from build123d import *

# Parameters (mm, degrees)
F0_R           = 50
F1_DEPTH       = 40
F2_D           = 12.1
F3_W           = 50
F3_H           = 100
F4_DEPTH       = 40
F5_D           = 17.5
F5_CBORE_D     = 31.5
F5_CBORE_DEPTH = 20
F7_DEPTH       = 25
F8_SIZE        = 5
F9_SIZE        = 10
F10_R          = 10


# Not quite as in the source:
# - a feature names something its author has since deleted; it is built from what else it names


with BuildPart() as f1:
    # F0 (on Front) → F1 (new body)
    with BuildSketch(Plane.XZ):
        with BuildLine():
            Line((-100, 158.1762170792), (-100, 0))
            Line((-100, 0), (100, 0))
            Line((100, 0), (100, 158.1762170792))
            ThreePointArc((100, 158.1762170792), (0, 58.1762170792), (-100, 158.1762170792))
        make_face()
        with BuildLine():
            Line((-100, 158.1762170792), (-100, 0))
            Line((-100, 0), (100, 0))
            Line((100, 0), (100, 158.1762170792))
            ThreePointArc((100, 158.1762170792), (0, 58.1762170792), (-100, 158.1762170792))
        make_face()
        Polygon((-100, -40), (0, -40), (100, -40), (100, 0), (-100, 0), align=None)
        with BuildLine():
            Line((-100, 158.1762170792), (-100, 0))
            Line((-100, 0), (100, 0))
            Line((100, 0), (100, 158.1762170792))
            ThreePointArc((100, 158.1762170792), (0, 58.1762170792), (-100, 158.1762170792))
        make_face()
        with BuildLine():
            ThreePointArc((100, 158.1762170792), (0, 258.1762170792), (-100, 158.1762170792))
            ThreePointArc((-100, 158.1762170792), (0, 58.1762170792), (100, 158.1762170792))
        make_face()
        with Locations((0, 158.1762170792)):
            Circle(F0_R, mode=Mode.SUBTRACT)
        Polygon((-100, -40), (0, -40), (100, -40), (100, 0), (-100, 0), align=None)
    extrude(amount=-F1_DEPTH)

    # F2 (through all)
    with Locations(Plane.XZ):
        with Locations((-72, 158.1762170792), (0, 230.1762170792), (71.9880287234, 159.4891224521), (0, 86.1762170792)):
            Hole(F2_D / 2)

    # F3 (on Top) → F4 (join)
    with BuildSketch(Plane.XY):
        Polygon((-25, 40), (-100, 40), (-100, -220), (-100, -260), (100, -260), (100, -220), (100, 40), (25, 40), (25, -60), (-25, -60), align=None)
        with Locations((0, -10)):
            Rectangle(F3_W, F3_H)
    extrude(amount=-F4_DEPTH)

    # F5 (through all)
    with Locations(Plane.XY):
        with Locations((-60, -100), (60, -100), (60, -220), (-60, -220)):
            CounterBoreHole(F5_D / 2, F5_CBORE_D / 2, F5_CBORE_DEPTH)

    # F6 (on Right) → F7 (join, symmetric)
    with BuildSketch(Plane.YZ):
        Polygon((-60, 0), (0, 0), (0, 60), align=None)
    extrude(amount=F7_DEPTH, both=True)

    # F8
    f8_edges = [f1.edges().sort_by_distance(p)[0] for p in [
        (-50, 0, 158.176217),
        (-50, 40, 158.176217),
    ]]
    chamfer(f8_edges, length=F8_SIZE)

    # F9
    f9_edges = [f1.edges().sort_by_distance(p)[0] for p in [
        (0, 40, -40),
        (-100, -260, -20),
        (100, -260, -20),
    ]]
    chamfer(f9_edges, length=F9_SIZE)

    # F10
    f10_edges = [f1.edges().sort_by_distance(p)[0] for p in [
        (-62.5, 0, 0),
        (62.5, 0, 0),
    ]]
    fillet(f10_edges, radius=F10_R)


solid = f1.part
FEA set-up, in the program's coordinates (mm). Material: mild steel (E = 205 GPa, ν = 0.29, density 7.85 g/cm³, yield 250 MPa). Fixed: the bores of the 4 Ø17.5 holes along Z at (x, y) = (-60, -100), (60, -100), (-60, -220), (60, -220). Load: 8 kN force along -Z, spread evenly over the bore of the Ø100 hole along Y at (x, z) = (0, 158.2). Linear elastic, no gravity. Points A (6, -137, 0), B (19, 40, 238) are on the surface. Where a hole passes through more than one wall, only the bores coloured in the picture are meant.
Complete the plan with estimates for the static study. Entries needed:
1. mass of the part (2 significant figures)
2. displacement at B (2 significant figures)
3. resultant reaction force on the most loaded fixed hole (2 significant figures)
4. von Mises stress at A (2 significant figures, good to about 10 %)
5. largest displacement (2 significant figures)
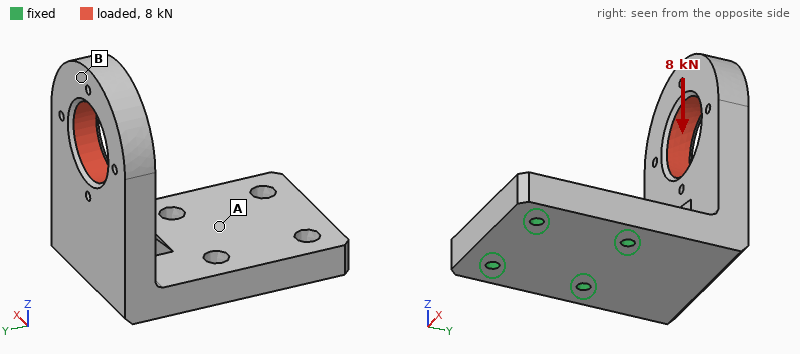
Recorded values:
31 kg
0.10 mm
8.2 kN
8.3 MPa
0.11 mm
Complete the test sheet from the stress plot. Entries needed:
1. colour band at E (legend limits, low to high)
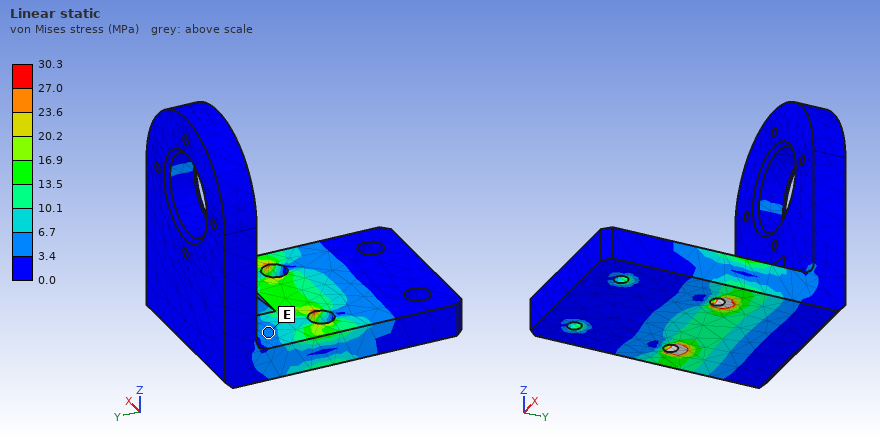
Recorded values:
3.4 to 6.7 MPa
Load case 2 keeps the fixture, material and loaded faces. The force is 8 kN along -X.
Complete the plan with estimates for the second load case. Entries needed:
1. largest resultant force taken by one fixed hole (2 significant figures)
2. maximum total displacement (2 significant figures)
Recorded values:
15 kN
90 µm
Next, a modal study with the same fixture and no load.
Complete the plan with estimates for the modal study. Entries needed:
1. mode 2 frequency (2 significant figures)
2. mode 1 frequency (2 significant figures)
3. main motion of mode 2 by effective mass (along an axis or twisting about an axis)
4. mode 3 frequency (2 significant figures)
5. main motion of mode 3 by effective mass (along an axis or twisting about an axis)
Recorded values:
590 Hz
330 Hz
along X
990 Hz
along Z
